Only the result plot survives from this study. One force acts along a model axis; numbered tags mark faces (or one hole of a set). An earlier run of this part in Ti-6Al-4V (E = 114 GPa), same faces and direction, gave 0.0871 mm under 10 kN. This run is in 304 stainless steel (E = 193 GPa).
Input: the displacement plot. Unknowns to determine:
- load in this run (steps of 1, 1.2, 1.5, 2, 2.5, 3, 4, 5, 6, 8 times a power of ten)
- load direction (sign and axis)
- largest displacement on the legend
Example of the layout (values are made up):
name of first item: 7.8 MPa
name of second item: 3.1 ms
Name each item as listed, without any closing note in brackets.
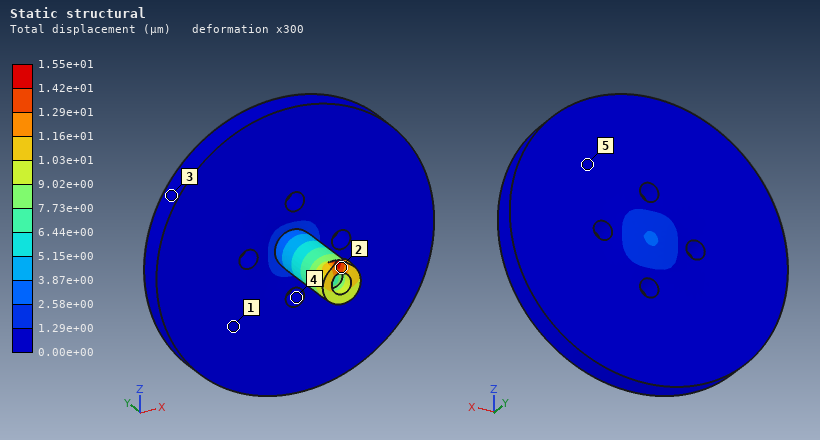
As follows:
load in this run: 3 kN
load direction: +Y
largest displacement on the legend: 1.55e+01 µm
